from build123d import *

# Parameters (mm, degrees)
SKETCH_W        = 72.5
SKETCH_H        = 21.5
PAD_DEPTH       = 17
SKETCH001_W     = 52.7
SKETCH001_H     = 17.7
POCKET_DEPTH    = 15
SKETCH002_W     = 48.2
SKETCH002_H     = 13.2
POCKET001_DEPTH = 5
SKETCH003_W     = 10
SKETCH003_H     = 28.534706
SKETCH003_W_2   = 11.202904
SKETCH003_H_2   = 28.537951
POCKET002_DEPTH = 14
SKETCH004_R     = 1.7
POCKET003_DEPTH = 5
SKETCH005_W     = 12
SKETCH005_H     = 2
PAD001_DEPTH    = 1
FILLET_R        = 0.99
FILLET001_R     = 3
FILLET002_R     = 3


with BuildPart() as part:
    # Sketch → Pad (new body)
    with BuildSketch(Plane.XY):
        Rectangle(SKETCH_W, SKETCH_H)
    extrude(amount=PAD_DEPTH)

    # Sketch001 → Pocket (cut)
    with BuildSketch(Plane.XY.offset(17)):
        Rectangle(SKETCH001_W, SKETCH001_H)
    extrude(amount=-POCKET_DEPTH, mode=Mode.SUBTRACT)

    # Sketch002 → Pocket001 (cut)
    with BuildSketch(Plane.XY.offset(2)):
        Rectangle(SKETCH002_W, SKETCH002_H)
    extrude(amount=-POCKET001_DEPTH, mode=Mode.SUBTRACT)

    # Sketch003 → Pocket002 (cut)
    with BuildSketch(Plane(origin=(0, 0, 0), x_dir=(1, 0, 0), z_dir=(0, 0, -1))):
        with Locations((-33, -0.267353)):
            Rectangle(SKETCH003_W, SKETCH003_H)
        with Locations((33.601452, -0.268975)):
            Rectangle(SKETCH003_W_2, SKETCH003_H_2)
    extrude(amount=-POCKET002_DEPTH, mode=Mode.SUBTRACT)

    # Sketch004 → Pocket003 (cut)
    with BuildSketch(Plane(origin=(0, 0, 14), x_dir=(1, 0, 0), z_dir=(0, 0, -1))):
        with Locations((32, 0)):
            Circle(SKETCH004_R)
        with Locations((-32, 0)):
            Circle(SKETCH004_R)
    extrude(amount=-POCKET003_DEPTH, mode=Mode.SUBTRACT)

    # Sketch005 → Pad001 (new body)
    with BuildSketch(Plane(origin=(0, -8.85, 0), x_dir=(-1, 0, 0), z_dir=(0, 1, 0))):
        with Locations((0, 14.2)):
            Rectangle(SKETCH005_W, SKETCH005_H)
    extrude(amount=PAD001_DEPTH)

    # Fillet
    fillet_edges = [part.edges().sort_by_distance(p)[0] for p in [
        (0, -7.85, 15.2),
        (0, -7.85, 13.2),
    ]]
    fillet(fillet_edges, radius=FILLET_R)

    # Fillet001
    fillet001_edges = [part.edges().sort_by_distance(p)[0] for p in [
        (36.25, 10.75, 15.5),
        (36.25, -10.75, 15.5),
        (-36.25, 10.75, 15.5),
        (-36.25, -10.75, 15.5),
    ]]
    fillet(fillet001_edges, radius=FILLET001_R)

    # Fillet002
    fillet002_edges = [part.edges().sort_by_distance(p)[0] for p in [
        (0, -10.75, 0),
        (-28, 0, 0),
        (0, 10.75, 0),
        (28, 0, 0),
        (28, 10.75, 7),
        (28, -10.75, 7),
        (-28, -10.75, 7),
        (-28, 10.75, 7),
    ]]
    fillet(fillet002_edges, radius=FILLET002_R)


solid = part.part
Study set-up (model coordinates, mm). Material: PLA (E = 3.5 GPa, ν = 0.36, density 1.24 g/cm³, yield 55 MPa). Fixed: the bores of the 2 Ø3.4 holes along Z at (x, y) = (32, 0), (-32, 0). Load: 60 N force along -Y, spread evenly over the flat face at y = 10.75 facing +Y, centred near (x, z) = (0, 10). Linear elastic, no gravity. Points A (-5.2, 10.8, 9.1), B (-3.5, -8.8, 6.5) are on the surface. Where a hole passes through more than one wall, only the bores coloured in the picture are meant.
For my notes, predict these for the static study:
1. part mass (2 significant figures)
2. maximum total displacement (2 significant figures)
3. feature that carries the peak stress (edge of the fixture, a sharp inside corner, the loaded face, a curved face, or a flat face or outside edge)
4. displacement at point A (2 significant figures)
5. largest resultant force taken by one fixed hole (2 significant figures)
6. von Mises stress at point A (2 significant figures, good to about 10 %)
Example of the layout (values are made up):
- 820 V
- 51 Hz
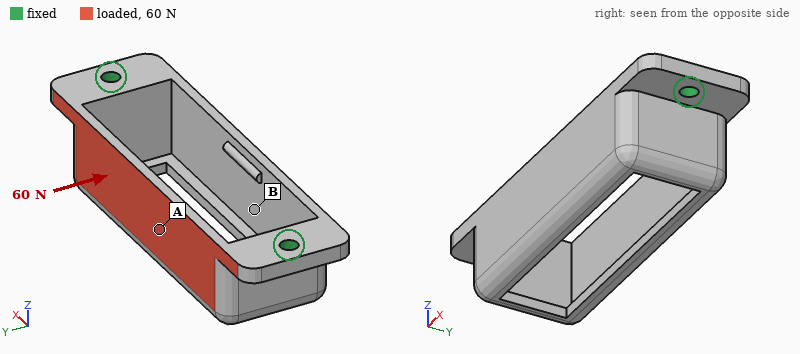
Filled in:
- 7.2 g
- 0.81 mm
- the loaded face
- 0.59 mm
- 36 N
- 10 MPa
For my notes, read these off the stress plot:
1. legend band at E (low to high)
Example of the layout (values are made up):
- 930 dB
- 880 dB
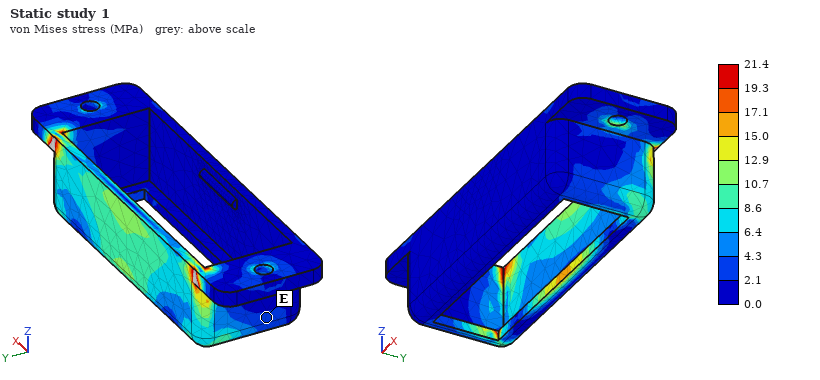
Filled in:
- 2.1 to 4.3 MPa
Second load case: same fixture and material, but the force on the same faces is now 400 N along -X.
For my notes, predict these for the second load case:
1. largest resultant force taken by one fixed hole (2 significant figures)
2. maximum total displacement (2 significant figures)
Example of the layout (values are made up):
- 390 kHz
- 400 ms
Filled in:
- 200 N
- 0.30 mm
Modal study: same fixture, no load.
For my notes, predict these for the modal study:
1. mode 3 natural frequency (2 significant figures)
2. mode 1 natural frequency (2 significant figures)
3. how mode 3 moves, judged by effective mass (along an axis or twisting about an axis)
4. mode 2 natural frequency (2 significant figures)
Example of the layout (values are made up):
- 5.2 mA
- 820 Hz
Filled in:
- 1700 Hz
- 1200 Hz
- twisting about X
- 1200 Hz
